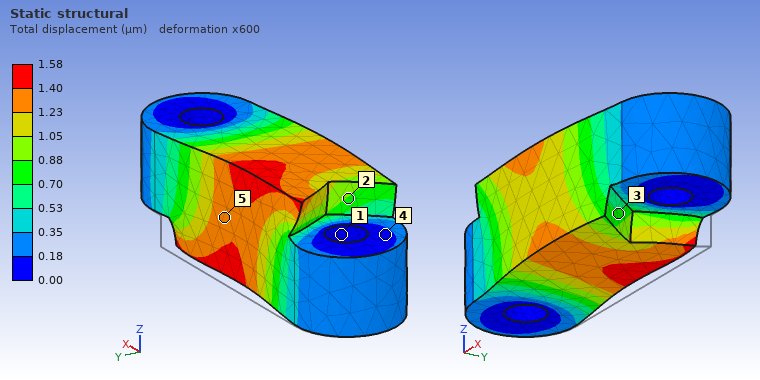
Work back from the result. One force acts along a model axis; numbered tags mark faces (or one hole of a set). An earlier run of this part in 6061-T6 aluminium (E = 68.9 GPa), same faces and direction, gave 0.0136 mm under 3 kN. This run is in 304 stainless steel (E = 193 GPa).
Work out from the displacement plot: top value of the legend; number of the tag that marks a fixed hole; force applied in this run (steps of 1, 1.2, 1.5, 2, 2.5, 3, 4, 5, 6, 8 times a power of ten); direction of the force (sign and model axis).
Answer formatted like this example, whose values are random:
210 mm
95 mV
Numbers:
1.58 µm
1
1 kN
-Y
